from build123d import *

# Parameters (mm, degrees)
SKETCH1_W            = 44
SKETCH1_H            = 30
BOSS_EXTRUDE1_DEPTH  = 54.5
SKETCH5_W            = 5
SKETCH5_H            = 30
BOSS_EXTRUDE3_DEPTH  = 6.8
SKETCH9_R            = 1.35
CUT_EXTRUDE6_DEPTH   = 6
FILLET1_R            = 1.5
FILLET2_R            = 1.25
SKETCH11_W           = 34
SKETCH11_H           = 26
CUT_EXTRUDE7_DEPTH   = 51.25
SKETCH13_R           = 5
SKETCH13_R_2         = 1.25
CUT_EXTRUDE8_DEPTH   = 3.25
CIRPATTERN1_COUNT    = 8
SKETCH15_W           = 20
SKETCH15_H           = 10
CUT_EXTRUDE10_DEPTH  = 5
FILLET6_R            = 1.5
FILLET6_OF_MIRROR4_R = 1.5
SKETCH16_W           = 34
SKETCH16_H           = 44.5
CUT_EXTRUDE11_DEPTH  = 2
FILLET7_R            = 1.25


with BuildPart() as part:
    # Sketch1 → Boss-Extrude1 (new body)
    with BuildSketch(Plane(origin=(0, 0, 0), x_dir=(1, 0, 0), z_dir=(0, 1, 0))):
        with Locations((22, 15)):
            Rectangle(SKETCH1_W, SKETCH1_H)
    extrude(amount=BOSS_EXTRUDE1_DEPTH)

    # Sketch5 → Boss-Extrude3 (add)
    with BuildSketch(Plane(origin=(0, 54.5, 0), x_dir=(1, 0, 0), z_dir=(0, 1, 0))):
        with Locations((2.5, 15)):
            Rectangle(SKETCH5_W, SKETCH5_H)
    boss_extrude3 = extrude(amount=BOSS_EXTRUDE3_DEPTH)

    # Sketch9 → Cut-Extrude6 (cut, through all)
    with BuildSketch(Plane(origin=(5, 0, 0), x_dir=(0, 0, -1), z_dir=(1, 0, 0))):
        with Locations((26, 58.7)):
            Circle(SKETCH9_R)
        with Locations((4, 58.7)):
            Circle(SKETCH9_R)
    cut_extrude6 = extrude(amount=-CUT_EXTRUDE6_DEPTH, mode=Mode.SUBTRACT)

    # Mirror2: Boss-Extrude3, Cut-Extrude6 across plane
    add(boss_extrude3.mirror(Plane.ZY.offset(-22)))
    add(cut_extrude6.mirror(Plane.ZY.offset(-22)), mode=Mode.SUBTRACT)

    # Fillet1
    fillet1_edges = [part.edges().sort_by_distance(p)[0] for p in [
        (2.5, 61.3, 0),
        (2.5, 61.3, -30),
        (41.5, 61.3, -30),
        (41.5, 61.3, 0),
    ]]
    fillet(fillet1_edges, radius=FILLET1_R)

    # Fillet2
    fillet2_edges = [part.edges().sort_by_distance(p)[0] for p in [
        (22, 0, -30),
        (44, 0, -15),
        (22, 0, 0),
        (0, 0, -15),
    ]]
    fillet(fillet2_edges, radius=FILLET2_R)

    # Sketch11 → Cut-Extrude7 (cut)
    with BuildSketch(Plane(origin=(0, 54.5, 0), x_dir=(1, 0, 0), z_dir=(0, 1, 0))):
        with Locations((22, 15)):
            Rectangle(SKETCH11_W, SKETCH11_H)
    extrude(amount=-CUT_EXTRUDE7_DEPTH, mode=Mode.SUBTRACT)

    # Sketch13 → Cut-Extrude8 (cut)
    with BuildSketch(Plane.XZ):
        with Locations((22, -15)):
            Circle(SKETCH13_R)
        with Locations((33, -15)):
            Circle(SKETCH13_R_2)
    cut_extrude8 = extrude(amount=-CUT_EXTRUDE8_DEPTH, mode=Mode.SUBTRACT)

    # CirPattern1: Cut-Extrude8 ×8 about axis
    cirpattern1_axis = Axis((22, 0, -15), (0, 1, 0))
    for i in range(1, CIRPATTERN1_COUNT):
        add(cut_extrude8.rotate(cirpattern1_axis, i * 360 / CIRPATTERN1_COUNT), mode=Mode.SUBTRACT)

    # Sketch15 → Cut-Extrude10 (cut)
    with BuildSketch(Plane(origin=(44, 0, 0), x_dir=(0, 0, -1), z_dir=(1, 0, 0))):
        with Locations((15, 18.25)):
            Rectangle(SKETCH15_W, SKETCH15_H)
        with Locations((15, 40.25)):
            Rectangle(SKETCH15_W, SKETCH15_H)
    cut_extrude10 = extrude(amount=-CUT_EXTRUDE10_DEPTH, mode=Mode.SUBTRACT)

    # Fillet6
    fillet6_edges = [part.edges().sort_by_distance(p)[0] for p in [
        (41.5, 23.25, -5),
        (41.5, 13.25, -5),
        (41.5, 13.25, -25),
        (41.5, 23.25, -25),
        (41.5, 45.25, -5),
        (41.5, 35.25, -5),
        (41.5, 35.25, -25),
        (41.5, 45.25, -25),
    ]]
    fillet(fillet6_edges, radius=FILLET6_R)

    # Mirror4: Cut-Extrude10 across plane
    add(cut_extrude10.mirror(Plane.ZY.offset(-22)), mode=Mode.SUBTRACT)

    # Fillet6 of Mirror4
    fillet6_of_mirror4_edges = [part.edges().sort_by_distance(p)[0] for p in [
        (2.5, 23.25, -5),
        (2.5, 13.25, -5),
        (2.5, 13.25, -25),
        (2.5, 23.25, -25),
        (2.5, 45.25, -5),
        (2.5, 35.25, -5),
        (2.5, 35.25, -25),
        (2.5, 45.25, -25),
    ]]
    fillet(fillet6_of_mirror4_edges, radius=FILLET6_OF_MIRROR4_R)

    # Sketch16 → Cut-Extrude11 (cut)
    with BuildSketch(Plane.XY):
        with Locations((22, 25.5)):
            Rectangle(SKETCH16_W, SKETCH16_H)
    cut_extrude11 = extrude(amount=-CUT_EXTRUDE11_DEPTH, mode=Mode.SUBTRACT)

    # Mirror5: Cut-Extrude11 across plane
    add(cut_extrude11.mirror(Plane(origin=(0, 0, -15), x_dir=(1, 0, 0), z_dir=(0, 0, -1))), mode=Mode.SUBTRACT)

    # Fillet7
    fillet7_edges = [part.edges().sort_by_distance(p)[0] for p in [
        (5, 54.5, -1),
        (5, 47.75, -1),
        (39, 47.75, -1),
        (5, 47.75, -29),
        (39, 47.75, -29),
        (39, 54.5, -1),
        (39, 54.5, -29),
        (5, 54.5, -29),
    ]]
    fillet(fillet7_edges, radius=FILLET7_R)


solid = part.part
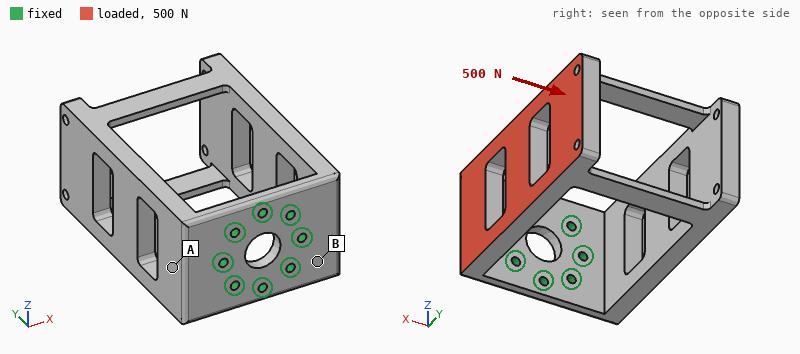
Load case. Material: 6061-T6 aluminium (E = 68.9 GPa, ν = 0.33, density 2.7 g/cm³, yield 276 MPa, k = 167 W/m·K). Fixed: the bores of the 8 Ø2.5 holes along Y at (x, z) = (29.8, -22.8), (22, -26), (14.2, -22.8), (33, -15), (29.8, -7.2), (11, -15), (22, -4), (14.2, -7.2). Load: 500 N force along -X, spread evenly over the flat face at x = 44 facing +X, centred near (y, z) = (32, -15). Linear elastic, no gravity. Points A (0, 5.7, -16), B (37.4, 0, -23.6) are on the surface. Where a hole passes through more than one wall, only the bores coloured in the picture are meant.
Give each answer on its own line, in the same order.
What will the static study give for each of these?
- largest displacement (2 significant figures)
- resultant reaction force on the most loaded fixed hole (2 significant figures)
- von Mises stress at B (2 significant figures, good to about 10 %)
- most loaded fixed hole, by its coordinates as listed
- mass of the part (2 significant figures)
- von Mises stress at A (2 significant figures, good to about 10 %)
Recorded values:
0.48 mm
450 N
83 MPa
(33, -15)
49 g
17 MPa
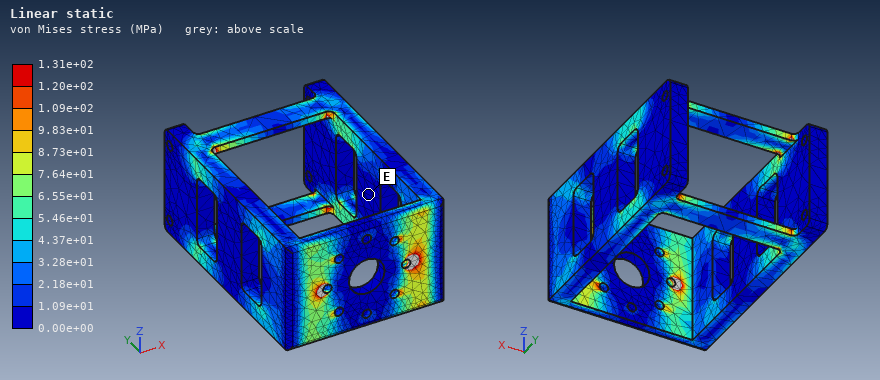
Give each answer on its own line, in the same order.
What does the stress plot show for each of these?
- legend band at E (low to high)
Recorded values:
0.00e+00 to 1.09e+01 MPa
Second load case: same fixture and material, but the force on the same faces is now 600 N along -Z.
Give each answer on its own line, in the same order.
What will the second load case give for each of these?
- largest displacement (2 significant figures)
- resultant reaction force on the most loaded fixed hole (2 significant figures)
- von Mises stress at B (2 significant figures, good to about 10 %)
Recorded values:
0.37 mm
810 N
59 MPa
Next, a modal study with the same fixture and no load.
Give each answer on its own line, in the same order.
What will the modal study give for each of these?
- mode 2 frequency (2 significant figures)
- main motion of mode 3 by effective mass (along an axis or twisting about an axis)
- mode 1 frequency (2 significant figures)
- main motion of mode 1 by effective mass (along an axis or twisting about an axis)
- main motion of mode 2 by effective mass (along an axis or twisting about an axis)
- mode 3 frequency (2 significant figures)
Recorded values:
1500 Hz
twisting about Y
910 Hz
along X
along Z
1900 Hz
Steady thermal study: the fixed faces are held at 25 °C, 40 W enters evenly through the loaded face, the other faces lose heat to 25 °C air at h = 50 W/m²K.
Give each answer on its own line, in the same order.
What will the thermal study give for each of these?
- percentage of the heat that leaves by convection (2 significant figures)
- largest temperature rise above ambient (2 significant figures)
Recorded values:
28 %
65 K
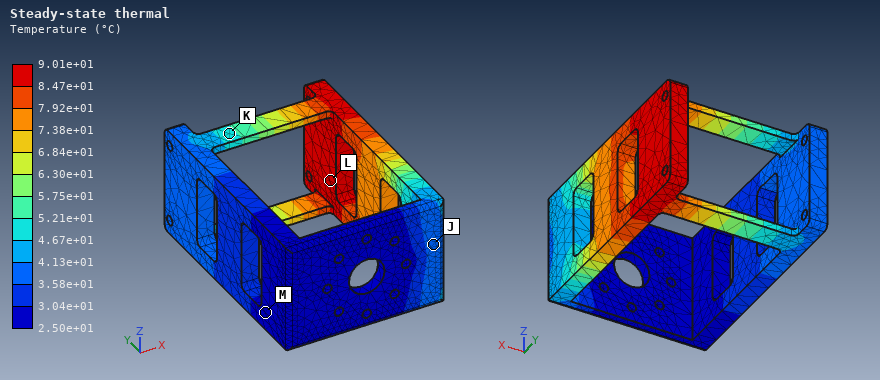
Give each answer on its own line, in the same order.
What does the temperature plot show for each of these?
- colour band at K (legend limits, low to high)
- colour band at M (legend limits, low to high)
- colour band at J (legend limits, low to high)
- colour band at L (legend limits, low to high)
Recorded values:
4.67e+01 to 5.21e+01 °C
2.50e+01 to 3.04e+01 °C
3.58e+01 to 4.13e+01 °C
8.47e+01 to 9.01e+01 °C
